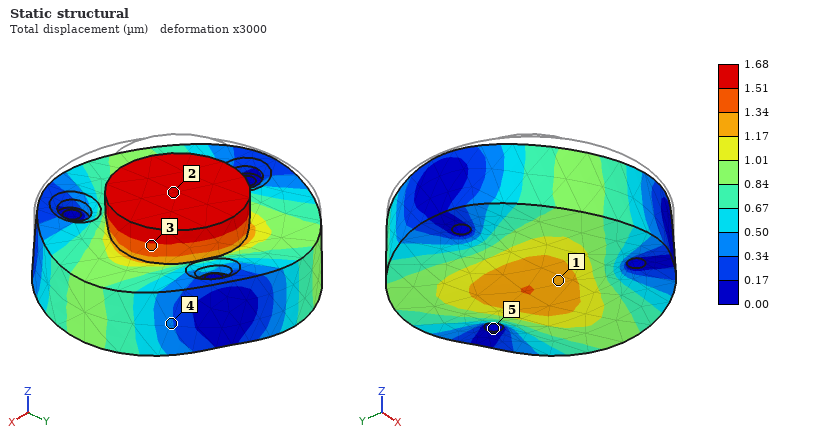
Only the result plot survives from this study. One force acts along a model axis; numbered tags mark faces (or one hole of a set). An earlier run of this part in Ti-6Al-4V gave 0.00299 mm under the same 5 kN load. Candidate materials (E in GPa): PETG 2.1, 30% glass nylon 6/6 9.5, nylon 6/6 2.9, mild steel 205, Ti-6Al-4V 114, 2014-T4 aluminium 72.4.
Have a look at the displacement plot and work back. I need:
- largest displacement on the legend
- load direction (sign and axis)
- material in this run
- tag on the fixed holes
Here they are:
1.68 µm
-Z
mild steel
5
